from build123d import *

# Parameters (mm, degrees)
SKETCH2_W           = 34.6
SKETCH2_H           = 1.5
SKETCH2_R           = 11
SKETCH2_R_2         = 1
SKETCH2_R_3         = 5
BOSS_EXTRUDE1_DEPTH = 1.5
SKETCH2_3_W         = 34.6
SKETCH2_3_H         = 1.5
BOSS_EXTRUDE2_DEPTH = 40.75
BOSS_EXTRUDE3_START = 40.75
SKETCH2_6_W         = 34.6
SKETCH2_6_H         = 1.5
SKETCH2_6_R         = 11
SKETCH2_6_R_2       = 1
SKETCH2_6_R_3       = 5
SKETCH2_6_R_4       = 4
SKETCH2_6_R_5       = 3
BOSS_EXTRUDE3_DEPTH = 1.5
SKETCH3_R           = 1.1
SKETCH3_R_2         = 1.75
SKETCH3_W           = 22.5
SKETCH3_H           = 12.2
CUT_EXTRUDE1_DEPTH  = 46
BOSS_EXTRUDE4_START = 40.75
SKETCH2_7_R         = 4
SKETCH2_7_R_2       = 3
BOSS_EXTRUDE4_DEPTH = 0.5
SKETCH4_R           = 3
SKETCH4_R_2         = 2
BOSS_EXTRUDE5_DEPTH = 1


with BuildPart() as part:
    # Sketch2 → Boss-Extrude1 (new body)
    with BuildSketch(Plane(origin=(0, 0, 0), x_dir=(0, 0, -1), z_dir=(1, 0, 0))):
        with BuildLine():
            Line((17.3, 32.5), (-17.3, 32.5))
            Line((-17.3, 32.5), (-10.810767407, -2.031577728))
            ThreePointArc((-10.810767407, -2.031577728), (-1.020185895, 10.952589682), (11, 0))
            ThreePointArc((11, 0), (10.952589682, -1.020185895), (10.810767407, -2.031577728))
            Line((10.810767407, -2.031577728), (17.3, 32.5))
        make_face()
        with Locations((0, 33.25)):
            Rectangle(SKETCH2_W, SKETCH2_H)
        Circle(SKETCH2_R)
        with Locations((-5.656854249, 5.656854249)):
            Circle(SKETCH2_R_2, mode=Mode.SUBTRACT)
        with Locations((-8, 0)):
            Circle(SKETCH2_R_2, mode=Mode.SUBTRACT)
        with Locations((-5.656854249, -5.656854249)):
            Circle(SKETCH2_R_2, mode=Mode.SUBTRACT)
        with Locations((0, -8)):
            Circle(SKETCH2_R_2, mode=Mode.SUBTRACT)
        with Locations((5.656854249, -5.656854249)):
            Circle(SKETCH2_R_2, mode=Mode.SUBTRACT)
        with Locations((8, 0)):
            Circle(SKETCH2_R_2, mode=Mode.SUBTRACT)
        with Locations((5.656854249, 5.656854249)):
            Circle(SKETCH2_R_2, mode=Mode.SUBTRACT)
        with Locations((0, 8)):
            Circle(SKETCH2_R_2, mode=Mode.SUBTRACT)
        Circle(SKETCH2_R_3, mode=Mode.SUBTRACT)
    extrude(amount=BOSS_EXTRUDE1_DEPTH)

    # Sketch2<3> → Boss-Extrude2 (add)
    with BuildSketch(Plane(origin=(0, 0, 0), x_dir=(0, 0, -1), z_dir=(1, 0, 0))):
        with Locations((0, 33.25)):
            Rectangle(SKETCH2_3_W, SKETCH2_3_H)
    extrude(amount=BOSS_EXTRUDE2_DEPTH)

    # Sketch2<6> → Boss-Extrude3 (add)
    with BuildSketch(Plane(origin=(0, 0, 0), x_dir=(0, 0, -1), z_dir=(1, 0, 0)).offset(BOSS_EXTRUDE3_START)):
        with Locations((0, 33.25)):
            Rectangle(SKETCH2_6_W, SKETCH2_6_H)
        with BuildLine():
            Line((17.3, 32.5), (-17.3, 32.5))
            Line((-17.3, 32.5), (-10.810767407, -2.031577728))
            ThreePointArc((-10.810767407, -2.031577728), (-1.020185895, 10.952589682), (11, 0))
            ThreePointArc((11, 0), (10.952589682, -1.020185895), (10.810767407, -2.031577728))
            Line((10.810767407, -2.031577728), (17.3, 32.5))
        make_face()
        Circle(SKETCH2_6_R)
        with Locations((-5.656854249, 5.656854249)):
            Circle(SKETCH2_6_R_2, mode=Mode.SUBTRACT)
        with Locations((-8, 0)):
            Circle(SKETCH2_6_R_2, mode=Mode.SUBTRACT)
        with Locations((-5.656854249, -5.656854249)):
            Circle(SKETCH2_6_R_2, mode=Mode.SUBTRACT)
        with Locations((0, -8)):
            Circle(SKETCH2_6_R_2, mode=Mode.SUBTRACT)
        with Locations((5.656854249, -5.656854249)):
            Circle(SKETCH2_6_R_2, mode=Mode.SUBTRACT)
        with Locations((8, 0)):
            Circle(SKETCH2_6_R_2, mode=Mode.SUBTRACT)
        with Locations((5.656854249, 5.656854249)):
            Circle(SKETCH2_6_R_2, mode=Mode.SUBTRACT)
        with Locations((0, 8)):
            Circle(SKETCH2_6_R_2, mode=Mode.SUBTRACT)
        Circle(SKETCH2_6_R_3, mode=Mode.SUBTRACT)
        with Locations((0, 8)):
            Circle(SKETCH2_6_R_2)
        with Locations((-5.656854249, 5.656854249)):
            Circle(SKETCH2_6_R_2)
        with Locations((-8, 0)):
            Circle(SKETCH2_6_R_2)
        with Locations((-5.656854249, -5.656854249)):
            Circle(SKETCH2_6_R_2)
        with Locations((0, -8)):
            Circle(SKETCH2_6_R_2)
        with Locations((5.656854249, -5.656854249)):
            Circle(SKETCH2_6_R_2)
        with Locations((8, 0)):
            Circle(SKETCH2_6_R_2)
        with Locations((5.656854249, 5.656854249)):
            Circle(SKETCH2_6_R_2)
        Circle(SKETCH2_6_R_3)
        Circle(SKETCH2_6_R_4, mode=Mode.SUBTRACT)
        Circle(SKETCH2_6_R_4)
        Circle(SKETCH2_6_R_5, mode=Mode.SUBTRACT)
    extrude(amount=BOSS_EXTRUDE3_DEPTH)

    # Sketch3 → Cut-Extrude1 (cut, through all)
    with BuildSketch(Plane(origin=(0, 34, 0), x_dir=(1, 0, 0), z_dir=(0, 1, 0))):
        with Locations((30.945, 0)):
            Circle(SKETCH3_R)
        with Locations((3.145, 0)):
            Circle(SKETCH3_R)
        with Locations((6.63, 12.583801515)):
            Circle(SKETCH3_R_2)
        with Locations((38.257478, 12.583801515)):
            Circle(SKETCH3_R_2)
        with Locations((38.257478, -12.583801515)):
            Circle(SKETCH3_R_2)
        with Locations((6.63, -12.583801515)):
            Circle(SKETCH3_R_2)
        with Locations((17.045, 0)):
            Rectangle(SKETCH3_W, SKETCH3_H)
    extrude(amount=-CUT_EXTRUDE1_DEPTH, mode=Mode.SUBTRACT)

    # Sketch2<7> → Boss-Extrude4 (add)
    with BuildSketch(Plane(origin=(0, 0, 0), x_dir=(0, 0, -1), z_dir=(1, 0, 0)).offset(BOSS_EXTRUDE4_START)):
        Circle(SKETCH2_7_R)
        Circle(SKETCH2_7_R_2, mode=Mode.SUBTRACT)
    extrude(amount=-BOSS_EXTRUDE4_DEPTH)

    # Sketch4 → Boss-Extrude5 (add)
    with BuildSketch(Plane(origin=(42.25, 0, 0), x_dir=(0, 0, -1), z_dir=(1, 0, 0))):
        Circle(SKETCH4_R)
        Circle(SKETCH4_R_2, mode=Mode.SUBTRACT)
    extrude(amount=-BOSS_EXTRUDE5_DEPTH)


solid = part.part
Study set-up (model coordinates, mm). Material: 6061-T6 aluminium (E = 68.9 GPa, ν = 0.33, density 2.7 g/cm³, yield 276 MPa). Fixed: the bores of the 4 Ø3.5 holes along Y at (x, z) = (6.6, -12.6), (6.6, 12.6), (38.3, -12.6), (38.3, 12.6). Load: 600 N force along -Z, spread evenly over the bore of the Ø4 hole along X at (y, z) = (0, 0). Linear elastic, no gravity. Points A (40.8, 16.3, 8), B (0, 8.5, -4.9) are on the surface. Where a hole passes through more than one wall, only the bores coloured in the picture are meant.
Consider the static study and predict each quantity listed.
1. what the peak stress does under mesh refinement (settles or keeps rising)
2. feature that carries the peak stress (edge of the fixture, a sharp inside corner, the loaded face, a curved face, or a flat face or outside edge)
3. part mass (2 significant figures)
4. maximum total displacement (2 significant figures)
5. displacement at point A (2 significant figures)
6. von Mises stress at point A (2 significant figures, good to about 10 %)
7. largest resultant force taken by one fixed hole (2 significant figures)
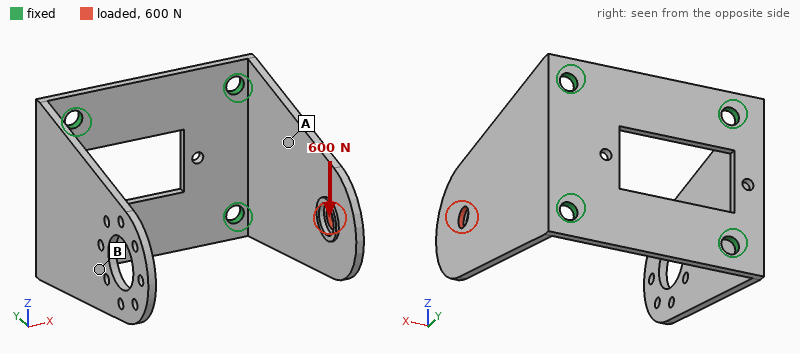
keeps rising
edge of the fixture
13 g
0.12 mm
0.050 mm
36 MPa
830 N
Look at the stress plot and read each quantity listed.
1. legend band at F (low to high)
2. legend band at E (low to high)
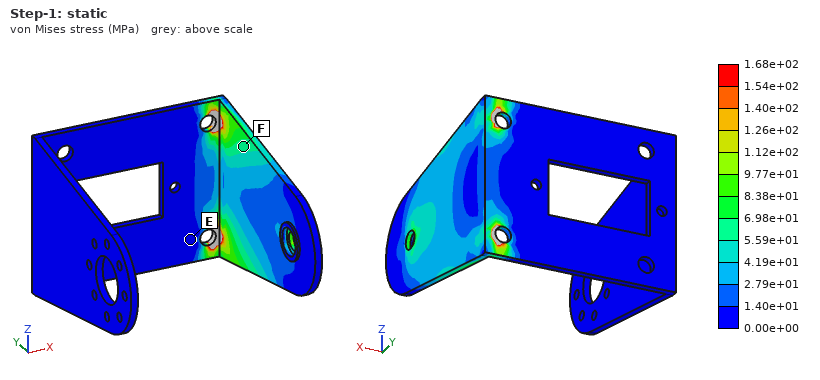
5.59e+01 to 6.98e+01 MPa
0.00e+00 to 1.40e+01 MPa
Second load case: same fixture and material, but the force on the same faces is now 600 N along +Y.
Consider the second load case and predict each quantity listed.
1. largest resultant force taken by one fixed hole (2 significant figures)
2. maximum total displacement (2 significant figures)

310 N
0.39 mm
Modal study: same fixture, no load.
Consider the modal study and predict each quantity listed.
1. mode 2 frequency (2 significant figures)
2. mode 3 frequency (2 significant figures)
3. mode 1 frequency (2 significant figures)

750 Hz
2900 Hz
740 Hz
